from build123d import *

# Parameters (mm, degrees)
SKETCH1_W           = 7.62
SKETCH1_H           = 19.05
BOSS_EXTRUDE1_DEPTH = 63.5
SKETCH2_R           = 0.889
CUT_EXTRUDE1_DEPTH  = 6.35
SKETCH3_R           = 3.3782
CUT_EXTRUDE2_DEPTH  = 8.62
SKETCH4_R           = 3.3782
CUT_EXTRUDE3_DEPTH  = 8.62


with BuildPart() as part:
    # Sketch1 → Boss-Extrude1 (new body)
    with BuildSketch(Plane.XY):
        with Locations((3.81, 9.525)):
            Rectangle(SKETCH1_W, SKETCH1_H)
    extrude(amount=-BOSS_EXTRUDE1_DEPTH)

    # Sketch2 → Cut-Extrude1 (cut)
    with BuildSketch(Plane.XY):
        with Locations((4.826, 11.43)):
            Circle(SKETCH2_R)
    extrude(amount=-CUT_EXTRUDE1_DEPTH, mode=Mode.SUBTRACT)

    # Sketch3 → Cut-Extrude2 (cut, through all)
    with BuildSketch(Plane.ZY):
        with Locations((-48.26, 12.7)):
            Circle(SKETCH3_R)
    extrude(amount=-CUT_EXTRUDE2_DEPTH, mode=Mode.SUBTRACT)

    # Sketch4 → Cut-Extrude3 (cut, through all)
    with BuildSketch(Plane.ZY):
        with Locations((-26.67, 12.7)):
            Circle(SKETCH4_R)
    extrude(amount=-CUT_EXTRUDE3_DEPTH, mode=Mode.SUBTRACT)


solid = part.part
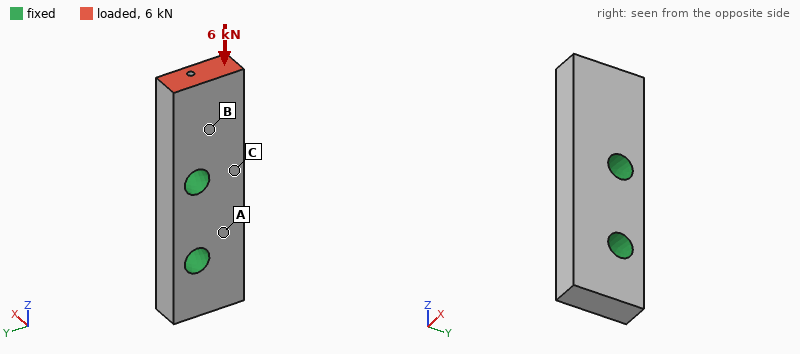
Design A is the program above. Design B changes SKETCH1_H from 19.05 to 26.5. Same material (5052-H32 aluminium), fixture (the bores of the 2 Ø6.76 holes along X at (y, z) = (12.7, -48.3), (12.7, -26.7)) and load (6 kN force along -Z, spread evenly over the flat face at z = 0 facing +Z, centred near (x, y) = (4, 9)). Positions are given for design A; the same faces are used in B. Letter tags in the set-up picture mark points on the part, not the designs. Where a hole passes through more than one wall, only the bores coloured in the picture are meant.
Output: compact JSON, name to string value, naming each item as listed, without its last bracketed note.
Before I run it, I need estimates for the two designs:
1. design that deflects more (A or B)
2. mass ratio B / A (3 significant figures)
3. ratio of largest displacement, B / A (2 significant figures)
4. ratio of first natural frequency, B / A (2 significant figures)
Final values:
{"design that deflects more": "A", "mass ratio B / A": "1.42", "ratio of largest displacement, B / A": "0.75", "ratio of first natural frequency, B / A": "0.94"}
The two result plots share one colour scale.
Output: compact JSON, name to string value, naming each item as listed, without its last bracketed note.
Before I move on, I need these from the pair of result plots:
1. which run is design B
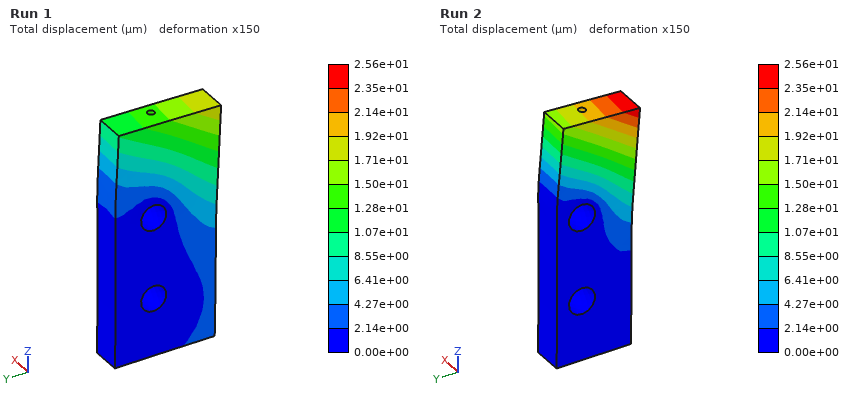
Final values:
{"which run is design B": "Run 1"}
